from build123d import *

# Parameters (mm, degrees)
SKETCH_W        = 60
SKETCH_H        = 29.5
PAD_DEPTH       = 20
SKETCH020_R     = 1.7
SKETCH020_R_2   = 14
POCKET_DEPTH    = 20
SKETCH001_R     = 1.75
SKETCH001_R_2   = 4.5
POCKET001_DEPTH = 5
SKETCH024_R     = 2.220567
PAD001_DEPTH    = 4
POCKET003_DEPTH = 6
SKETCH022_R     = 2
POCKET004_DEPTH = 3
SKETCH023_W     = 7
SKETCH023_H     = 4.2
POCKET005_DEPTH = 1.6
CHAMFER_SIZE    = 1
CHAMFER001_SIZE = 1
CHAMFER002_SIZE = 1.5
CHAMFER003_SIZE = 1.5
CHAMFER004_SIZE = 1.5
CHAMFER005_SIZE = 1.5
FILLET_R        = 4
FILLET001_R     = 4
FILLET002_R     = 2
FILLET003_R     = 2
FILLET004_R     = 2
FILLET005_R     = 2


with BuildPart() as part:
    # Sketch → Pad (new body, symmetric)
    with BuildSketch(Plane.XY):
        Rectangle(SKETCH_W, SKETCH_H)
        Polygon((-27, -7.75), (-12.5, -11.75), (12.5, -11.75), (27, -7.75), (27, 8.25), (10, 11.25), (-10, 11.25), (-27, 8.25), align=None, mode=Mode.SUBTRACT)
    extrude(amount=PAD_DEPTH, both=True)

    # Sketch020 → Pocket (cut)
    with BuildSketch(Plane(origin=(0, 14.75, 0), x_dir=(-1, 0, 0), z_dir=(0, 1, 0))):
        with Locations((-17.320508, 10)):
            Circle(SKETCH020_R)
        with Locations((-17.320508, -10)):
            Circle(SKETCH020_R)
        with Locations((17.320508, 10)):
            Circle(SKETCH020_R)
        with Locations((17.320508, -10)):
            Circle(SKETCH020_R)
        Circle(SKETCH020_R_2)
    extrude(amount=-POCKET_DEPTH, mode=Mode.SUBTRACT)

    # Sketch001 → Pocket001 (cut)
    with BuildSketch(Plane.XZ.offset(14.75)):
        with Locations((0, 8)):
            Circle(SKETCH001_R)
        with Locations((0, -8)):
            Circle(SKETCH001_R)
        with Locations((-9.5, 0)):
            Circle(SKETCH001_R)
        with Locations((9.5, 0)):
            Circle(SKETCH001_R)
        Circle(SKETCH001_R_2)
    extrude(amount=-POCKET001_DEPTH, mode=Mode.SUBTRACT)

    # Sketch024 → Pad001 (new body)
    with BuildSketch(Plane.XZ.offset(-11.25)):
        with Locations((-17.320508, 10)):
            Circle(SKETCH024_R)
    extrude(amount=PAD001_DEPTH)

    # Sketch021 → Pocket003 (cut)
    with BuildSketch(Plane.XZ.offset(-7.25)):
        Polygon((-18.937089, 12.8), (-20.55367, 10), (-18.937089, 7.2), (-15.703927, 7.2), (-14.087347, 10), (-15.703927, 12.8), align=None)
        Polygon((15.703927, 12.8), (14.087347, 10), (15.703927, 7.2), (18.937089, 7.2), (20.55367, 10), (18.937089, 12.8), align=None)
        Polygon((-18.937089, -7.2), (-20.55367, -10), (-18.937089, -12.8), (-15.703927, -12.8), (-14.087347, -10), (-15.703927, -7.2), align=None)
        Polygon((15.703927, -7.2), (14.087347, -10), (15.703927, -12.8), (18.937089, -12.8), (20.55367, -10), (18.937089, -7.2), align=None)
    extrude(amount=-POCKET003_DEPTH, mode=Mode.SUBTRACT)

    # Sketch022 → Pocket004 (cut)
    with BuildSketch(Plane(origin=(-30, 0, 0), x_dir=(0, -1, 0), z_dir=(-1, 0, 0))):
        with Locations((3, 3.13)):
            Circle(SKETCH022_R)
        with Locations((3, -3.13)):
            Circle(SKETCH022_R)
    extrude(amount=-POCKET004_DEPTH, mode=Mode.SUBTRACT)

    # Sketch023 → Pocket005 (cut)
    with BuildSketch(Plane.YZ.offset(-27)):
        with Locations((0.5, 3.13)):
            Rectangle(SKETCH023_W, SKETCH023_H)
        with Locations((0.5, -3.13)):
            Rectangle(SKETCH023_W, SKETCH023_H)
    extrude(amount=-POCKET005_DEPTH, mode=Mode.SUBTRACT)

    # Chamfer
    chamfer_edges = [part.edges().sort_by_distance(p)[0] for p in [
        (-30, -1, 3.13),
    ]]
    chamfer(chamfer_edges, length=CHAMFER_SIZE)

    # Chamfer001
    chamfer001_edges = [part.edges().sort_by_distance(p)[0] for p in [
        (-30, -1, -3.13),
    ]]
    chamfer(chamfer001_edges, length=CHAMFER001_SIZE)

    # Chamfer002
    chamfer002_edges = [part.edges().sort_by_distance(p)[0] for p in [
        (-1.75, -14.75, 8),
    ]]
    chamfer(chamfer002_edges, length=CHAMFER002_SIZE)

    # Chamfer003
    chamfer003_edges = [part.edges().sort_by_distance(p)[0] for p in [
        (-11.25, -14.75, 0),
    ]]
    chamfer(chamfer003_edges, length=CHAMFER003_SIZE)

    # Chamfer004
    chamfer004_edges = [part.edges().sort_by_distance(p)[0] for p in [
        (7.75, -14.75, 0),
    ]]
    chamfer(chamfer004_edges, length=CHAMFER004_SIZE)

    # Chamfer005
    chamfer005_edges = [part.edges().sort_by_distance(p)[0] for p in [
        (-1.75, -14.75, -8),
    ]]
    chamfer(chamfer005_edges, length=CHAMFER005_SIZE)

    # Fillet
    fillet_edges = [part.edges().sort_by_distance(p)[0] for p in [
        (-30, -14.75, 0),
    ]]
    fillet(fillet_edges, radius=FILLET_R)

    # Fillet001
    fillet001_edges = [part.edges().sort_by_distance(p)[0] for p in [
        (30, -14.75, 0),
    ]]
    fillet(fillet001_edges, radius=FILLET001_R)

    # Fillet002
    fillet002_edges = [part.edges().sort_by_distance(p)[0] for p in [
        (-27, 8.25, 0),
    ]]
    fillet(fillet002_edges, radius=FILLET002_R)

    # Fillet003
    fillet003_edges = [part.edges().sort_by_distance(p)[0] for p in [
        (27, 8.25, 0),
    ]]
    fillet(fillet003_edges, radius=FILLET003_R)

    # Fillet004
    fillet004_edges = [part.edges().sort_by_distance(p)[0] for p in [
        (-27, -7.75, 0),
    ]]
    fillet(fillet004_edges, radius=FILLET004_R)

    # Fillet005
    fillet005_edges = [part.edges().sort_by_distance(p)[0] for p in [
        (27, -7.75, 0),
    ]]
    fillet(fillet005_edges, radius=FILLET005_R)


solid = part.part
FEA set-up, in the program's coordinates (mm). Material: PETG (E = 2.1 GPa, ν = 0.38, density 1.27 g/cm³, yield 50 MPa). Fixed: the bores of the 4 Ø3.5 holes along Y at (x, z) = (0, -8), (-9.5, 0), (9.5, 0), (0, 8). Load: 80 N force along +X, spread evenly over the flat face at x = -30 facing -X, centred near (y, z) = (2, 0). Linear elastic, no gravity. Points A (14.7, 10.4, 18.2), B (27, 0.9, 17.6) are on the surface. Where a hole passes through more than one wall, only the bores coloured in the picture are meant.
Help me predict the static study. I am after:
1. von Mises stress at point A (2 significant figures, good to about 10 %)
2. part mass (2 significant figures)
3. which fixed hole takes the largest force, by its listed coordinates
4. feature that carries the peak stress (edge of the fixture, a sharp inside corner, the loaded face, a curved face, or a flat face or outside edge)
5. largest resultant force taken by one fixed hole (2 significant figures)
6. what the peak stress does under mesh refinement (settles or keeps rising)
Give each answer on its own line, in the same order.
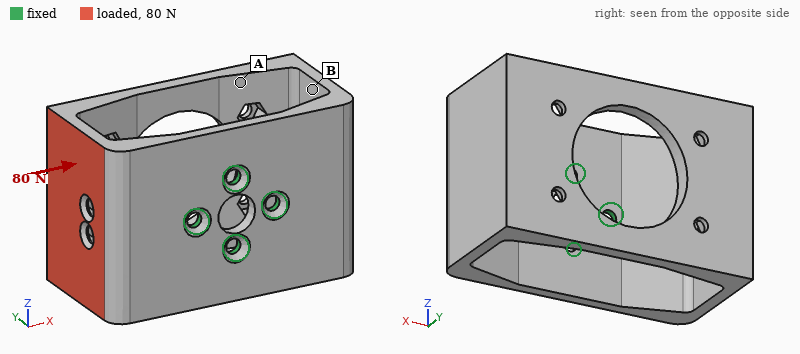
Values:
2.7 MPa
28 g
(-9.5, 0)
edge of the fixture
74 N
keeps rising
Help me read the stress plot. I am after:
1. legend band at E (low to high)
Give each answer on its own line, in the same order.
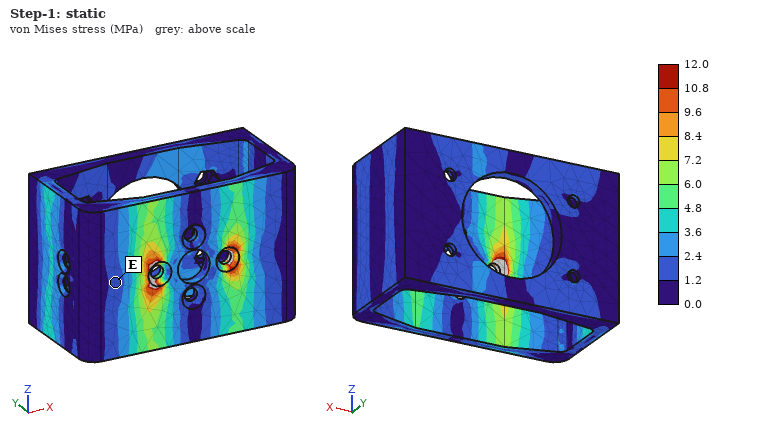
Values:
1.2 to 2.4 MPa
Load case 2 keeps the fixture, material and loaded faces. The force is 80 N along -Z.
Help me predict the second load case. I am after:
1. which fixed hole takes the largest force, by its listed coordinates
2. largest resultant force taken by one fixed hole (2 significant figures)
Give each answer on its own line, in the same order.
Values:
(-9.5, 0)
95 N
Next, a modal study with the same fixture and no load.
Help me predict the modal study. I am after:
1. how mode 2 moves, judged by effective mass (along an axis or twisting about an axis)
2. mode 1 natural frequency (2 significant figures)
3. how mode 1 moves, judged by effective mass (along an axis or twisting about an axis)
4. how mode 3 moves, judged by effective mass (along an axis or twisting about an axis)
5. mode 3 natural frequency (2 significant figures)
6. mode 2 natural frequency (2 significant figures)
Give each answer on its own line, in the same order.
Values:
along Z
320 Hz
along X
along Y
540 Hz
380 Hz
